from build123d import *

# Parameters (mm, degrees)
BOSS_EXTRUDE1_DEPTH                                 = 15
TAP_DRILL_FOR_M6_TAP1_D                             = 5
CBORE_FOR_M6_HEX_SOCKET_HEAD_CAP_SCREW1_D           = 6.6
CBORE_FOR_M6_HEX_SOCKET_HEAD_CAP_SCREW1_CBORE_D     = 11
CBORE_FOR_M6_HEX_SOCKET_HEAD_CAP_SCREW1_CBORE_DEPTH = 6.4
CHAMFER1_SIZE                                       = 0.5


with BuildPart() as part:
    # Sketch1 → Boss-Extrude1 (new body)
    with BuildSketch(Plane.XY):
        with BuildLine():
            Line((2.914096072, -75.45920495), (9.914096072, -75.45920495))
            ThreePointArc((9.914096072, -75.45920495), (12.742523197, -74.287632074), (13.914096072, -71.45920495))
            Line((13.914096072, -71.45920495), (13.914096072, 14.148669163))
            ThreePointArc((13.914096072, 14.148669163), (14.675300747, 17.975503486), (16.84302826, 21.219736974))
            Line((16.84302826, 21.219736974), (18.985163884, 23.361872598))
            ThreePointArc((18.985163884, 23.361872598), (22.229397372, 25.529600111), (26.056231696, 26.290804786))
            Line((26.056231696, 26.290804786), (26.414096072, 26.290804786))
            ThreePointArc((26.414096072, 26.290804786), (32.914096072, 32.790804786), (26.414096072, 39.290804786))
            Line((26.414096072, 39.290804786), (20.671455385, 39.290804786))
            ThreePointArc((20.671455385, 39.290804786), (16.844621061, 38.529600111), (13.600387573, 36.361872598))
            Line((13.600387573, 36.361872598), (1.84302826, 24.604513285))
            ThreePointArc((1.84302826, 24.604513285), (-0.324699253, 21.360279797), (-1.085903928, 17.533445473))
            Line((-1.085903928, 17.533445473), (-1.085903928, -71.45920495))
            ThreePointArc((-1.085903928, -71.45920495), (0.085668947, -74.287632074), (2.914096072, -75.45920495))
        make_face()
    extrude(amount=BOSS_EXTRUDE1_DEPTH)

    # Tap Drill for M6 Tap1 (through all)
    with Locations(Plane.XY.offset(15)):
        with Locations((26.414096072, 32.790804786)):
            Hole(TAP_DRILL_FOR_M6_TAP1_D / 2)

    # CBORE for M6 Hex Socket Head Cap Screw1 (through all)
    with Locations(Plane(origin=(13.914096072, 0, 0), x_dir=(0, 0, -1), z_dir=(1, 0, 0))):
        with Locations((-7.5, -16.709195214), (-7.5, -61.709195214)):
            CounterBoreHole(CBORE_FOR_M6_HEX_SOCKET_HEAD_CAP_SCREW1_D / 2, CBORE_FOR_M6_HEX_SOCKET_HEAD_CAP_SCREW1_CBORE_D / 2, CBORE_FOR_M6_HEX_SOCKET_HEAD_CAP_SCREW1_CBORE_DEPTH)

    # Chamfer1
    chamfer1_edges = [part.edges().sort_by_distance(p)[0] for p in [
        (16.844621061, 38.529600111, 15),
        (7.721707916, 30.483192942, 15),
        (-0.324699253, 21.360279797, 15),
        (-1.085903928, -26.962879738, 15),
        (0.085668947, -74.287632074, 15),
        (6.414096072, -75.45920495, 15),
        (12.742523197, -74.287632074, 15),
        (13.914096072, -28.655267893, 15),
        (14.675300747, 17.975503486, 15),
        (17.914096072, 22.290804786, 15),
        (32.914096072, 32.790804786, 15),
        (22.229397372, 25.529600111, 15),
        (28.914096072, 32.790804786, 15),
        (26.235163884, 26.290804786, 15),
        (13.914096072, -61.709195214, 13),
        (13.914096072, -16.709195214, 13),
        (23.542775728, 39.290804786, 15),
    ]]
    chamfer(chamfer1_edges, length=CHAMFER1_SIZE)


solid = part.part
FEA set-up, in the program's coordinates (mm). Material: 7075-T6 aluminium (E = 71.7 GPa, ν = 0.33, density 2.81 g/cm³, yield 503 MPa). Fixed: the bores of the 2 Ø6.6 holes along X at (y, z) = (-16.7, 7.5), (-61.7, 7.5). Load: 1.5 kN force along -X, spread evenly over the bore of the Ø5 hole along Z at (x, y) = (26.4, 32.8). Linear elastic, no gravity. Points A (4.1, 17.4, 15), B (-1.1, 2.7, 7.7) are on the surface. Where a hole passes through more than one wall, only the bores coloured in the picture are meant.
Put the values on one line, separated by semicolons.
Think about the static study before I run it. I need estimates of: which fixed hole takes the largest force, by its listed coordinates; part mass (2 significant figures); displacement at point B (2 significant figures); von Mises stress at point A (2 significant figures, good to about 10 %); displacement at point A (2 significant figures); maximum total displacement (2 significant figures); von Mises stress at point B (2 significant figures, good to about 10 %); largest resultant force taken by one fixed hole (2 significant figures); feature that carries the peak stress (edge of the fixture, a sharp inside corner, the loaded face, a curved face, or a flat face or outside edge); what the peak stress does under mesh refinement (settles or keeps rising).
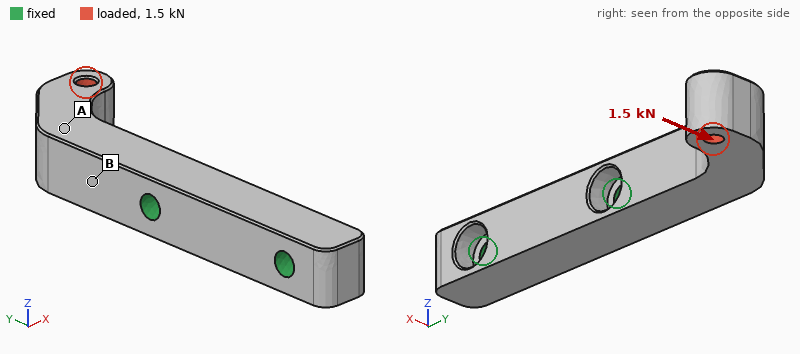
(-16.7, 7.5); 71 g; 0.089 mm; 30 MPa; 0.19 mm; 0.42 mm; 80 MPa; 2.3 kN; edge of the fixture; keeps rising
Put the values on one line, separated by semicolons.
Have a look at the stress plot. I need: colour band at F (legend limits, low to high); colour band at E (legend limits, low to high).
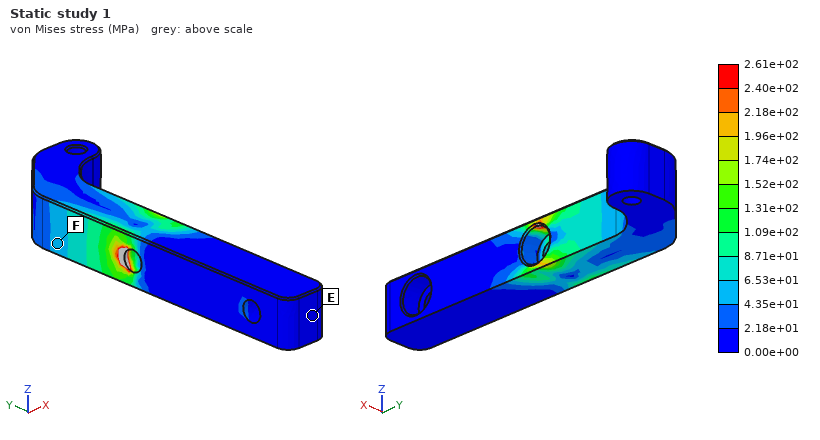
4.35e+01 to 6.53e+01 MPa; 0.00e+00 to 2.18e+01 MPa
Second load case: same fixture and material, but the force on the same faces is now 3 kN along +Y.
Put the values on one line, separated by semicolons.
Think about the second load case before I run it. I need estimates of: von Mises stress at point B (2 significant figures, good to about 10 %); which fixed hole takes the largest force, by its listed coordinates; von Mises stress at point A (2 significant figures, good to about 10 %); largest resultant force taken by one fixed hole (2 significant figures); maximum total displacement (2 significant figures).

94 MPa; (-16.7, 7.5); 48 MPa; 1.9 kN; 0.53 mm
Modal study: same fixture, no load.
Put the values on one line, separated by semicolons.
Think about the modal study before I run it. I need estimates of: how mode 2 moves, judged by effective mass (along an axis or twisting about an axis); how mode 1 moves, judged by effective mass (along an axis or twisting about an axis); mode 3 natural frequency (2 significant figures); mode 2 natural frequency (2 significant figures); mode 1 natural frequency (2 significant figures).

along Z; along X; 8100 Hz; 2700 Hz; 2600 Hz
